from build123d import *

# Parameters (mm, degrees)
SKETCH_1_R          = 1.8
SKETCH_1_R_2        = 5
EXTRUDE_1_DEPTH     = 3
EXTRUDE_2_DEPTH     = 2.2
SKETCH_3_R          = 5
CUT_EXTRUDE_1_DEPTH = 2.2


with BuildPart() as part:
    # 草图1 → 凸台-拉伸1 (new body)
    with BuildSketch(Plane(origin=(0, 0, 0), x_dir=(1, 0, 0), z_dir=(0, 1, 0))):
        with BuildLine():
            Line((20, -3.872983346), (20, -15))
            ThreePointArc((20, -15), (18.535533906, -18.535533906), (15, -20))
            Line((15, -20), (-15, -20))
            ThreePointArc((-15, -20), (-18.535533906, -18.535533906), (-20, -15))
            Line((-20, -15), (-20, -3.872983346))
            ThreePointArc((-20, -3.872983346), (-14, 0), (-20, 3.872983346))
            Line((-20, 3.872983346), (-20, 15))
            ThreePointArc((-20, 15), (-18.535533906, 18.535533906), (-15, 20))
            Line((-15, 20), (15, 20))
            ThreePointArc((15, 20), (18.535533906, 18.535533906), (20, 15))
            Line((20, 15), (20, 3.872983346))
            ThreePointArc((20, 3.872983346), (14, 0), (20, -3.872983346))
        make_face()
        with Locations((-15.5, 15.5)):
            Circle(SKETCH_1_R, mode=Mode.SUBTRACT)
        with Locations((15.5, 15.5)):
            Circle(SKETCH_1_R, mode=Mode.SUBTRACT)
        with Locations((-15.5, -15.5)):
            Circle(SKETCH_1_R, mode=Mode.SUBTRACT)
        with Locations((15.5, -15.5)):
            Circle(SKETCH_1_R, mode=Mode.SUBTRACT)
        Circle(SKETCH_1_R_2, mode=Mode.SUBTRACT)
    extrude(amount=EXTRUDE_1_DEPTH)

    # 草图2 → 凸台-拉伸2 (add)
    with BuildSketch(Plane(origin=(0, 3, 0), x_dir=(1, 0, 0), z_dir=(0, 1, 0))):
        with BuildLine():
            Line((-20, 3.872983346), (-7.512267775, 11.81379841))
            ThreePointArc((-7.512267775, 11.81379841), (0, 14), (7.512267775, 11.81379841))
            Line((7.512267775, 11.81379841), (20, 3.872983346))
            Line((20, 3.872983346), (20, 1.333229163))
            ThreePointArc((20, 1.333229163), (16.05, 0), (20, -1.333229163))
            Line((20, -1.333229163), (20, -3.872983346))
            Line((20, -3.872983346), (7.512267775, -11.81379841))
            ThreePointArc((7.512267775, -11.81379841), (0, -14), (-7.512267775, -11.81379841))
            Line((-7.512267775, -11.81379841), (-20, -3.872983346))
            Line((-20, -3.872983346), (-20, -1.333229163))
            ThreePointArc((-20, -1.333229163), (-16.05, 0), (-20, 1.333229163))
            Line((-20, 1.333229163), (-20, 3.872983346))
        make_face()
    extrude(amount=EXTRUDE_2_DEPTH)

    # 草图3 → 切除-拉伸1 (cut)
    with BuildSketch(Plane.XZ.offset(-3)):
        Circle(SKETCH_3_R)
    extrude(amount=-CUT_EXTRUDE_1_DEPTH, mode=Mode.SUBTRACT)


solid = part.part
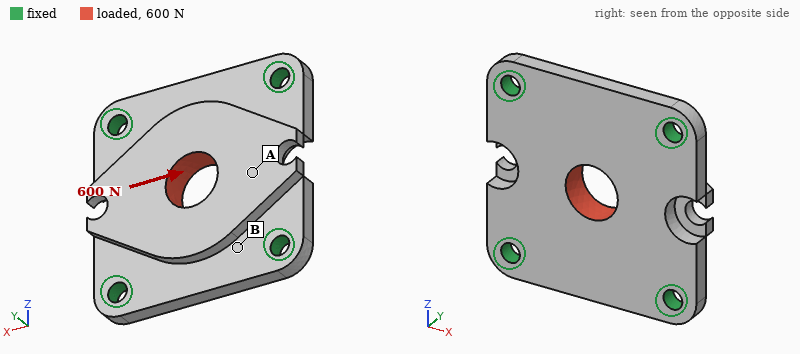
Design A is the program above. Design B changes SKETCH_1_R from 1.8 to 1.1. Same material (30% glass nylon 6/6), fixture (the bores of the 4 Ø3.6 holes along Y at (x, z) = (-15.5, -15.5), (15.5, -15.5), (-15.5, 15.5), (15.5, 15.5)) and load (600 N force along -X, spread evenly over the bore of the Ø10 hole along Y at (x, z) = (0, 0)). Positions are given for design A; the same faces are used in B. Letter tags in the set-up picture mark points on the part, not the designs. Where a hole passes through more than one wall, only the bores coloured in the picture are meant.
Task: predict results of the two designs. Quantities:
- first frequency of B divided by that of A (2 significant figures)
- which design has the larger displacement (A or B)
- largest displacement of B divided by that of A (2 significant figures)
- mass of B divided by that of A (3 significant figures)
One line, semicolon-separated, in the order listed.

0.88; B; 1.1; 1.01
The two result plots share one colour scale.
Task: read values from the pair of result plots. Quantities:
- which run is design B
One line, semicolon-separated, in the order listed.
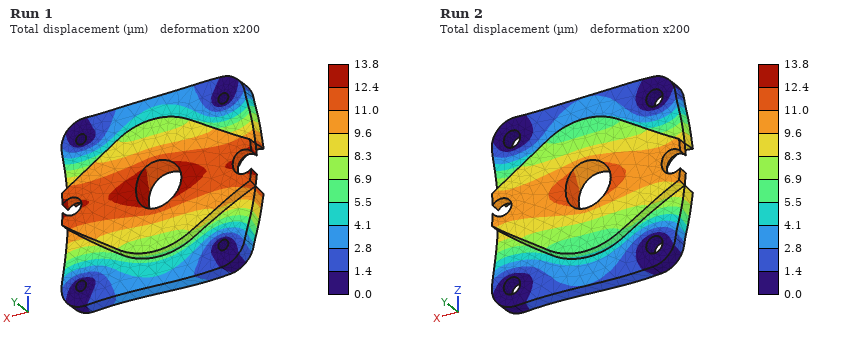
Run 1
